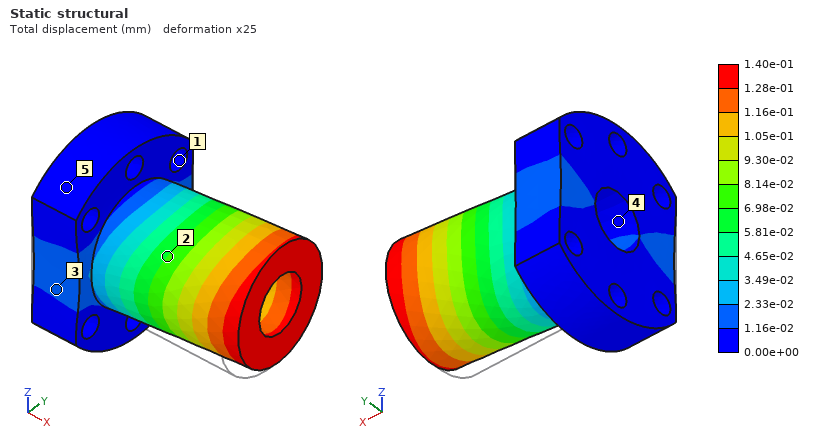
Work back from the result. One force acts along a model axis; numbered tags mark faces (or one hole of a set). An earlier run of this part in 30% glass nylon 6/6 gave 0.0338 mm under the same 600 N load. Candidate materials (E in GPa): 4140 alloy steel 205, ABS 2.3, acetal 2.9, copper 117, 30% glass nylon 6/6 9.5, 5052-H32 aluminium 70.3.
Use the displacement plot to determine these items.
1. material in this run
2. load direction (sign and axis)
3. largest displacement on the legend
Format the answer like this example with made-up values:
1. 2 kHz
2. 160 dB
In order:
1. ABS
2. +Y
3. 1.40e-01 mm
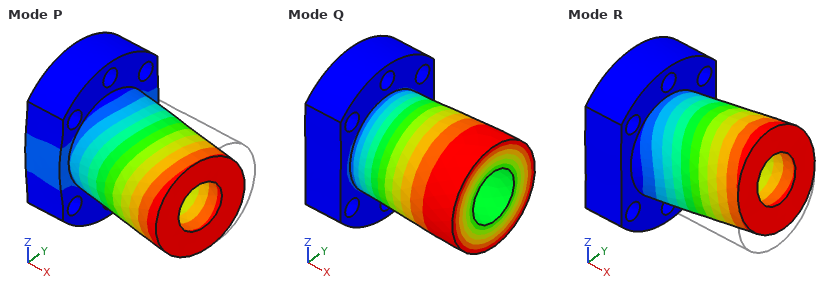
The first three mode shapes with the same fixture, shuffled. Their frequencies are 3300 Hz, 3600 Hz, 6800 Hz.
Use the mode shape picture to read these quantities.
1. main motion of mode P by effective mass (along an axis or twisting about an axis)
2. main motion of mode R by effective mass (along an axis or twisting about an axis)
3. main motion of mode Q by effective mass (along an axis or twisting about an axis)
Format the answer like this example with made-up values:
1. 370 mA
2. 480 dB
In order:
1. along Y
2. along Z
3. twisting about X
